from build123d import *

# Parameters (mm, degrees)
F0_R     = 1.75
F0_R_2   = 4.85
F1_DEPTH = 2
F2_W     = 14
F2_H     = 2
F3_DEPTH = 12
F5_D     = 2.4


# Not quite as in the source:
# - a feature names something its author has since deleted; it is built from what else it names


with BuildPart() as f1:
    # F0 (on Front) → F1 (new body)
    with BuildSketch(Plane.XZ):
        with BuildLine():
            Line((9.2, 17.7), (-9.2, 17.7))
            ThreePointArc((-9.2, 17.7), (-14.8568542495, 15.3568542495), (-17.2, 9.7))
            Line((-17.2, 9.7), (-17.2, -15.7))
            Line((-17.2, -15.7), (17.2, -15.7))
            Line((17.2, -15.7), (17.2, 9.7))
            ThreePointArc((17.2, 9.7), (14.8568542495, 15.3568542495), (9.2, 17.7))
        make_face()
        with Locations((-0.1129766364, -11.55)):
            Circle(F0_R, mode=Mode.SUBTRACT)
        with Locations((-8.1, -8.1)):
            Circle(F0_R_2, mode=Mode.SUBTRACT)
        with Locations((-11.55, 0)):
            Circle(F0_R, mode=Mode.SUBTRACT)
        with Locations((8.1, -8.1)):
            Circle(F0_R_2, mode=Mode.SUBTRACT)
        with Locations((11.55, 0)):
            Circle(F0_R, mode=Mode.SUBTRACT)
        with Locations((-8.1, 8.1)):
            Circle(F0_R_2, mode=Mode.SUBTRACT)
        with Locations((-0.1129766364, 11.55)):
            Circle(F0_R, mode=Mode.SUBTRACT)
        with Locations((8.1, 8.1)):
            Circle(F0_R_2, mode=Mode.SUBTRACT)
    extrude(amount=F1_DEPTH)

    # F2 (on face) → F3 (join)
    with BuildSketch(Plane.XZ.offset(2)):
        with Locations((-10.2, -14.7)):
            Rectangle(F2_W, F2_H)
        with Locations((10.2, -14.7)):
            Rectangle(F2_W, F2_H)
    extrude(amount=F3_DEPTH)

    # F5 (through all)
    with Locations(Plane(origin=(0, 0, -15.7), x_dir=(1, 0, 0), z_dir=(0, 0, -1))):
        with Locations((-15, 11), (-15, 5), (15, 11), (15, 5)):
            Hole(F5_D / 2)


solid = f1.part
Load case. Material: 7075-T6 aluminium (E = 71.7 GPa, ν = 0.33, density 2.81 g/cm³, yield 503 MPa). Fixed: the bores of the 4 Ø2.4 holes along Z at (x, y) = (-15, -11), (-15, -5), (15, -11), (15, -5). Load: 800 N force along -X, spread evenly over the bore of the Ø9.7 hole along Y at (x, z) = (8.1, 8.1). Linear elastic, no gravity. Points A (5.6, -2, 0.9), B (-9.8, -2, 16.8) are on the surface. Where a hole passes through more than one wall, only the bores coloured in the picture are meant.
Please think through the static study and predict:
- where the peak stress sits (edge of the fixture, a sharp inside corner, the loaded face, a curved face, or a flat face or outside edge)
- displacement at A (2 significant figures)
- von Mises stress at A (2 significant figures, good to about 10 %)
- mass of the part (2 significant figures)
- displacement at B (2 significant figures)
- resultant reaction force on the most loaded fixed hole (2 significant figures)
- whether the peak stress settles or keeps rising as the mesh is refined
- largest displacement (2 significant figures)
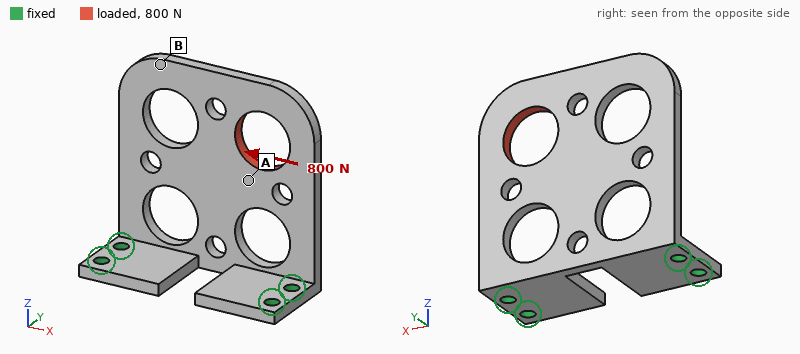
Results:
edge of the fixture
0.076 mm
60 MPa
6.2 g
0.13 mm
800 N
keeps rising
0.15 mm
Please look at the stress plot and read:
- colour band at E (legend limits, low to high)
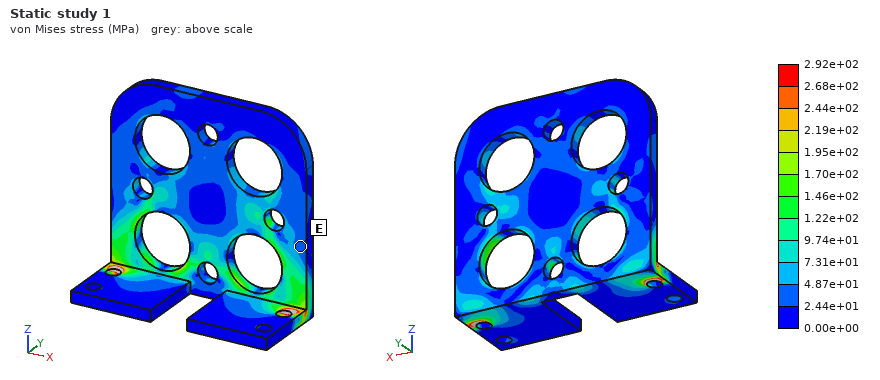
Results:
2.44e+01 to 4.87e+01 MPa
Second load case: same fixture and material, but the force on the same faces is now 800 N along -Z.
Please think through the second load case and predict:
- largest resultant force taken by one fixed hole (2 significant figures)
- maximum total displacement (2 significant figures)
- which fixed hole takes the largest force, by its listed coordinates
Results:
690 N
0.21 mm
(15, -5)
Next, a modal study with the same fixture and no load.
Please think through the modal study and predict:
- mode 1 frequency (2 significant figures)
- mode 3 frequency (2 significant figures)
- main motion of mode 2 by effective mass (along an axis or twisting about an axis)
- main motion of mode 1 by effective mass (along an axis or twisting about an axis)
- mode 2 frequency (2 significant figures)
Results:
1100 Hz
7200 Hz
twisting about Z
along Y
3200 Hz
